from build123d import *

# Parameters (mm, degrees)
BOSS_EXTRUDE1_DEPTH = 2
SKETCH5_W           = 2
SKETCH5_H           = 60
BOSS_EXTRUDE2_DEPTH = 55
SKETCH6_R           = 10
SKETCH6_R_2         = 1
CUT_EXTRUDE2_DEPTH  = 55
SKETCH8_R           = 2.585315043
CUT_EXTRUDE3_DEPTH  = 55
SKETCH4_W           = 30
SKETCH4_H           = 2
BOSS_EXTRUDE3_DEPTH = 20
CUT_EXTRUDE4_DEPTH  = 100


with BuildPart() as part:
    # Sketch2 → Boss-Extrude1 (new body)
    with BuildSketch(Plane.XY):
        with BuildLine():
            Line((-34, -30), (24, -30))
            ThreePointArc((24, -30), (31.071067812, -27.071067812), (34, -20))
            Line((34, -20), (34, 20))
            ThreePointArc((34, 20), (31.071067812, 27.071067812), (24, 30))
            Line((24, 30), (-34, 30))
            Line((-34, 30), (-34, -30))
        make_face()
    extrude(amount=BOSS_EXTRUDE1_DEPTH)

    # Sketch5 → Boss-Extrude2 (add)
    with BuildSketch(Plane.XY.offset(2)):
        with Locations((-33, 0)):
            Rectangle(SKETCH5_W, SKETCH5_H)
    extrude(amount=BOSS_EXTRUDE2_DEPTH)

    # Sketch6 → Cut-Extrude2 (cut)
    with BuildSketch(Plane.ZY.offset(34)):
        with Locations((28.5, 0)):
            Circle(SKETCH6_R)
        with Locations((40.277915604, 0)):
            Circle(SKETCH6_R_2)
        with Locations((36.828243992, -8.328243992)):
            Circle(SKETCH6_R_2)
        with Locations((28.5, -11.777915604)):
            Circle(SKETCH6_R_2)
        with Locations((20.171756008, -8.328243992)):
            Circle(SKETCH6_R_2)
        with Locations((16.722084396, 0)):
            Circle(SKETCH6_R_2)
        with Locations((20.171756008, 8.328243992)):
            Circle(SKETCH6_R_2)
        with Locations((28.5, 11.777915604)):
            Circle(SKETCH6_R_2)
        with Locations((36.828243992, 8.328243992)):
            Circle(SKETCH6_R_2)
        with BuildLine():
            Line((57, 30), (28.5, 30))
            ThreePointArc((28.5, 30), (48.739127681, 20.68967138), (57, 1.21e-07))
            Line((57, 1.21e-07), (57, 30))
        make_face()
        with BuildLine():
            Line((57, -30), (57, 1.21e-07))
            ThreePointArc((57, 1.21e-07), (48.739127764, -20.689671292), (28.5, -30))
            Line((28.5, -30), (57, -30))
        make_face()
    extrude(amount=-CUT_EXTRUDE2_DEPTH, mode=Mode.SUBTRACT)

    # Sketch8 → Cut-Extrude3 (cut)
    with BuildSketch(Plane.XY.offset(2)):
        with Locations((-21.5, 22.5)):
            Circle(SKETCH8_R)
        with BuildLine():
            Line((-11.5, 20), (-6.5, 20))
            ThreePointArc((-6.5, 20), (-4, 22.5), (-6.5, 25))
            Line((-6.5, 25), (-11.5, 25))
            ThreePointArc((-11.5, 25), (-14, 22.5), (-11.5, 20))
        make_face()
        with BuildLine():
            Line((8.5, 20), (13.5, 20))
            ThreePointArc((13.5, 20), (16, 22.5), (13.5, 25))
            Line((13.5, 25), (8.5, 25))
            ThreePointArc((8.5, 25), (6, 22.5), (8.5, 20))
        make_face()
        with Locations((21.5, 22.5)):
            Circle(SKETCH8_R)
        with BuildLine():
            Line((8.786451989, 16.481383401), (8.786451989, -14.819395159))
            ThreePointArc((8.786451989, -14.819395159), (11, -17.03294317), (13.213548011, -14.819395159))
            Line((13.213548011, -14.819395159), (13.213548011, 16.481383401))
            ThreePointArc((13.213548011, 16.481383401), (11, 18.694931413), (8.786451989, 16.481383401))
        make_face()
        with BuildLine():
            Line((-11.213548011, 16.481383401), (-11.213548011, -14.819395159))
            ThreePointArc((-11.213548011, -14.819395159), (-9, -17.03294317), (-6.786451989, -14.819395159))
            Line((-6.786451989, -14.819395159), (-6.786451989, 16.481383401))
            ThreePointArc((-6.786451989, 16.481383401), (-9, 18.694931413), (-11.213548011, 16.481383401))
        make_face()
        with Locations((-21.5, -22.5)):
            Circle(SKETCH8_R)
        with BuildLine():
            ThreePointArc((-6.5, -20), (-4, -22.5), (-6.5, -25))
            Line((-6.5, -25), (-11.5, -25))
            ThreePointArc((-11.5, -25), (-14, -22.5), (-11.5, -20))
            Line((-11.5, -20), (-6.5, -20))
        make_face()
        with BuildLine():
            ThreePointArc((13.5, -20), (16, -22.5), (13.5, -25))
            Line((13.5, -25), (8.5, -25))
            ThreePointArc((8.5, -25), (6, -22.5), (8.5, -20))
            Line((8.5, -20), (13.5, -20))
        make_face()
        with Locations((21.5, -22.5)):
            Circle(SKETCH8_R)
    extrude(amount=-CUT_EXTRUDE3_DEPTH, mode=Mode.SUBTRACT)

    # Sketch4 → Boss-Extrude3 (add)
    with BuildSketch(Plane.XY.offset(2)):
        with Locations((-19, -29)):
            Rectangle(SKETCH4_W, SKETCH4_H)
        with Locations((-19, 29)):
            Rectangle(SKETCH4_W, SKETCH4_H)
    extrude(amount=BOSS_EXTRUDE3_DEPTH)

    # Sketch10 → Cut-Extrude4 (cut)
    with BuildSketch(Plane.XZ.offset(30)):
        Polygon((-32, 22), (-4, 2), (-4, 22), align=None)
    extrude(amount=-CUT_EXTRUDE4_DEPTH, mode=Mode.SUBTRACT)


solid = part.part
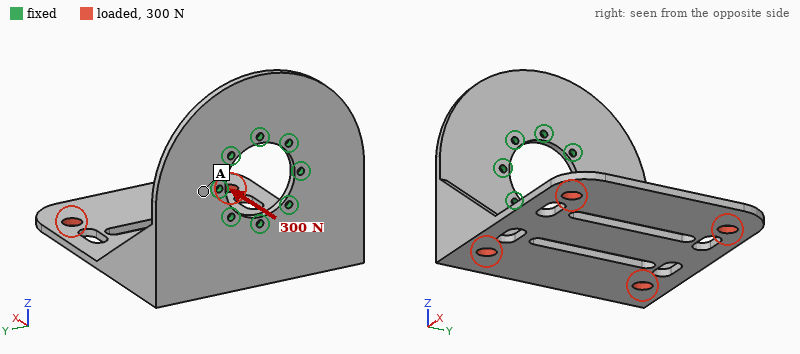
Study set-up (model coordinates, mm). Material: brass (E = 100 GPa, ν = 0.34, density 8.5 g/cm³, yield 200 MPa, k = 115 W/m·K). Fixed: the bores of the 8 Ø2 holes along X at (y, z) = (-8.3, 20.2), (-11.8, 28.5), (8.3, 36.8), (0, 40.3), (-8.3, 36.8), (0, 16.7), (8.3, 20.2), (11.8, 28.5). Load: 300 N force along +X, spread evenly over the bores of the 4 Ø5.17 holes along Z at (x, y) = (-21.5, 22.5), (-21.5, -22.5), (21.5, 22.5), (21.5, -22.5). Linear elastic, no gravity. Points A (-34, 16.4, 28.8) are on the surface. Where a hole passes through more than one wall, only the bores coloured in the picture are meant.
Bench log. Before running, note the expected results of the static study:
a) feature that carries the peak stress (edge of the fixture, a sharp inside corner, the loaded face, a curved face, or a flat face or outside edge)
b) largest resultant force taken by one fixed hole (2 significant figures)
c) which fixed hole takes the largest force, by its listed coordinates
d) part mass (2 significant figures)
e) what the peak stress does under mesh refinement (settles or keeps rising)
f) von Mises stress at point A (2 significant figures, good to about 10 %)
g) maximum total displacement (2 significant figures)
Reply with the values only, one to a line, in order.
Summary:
edge of the fixture
260 N
(0, 16.7)
110 g
keeps rising
20 MPa
0.51 mm
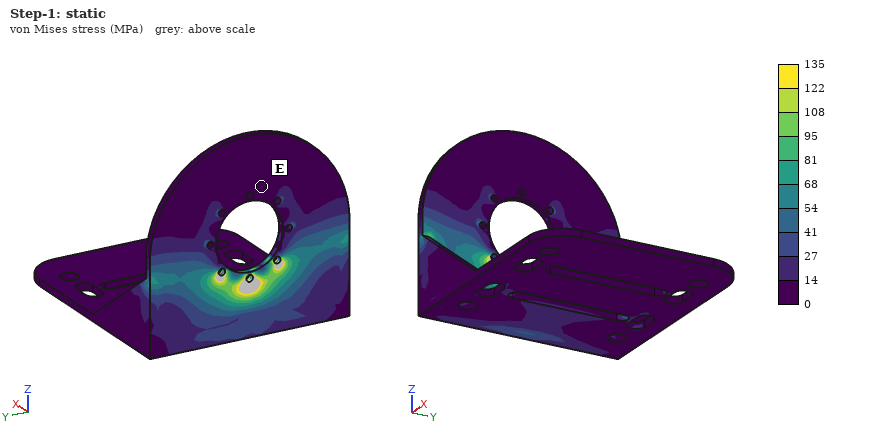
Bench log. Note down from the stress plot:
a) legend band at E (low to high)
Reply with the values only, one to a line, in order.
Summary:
0 to 14 MPa
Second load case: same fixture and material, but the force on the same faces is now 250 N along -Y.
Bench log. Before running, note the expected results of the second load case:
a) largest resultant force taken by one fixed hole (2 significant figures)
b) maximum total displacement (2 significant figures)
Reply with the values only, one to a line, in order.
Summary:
260 N
0.86 mm
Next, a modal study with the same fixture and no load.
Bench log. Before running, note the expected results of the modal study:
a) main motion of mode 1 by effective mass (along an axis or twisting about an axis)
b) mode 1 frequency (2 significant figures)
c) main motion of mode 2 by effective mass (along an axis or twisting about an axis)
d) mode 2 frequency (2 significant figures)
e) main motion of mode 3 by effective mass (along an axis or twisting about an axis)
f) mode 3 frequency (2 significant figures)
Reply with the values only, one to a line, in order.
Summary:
along Z
270 Hz
along Y
380 Hz
along X
830 Hz
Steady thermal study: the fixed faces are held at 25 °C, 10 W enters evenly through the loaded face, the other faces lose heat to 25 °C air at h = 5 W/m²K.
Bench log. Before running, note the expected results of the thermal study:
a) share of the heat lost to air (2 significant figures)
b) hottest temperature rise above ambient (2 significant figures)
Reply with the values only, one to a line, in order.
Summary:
14 %
52 K
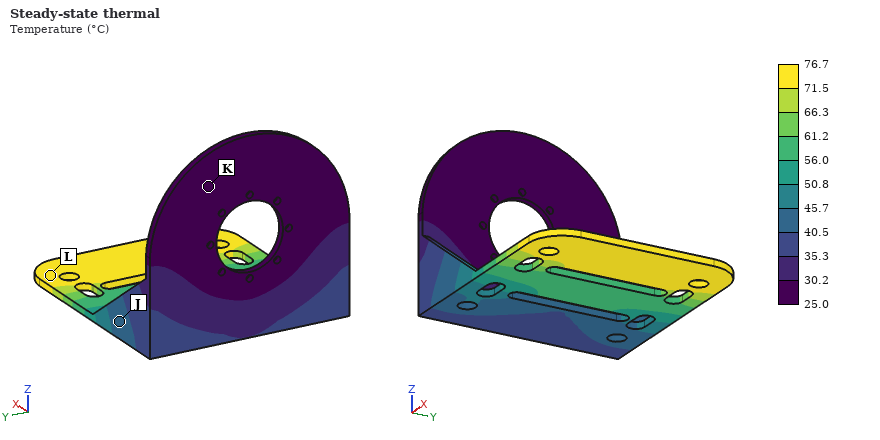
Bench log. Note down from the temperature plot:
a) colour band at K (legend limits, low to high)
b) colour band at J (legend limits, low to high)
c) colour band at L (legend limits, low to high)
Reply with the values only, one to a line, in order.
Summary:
25.0 to 30.2 °C
40.5 to 45.7 °C
71.5 to 76.7 °C
